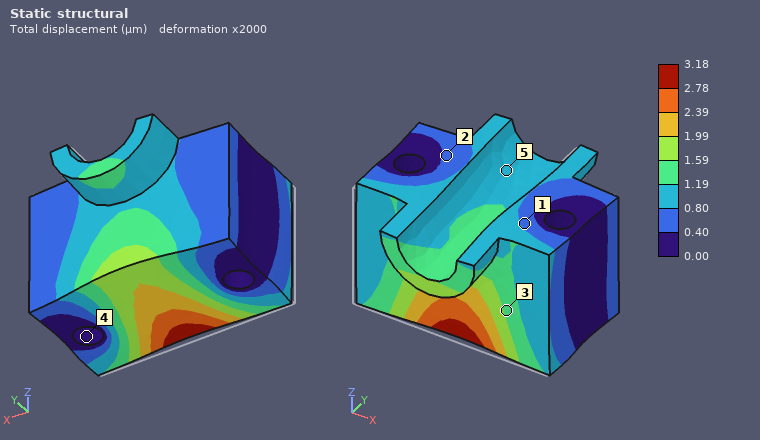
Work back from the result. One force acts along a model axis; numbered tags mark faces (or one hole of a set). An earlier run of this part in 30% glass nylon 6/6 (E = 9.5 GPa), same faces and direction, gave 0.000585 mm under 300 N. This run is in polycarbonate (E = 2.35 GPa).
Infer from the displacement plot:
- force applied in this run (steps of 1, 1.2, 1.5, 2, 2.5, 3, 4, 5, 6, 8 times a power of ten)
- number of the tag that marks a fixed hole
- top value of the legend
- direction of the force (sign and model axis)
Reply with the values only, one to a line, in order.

400 N
4
3.18 µm
+Y
